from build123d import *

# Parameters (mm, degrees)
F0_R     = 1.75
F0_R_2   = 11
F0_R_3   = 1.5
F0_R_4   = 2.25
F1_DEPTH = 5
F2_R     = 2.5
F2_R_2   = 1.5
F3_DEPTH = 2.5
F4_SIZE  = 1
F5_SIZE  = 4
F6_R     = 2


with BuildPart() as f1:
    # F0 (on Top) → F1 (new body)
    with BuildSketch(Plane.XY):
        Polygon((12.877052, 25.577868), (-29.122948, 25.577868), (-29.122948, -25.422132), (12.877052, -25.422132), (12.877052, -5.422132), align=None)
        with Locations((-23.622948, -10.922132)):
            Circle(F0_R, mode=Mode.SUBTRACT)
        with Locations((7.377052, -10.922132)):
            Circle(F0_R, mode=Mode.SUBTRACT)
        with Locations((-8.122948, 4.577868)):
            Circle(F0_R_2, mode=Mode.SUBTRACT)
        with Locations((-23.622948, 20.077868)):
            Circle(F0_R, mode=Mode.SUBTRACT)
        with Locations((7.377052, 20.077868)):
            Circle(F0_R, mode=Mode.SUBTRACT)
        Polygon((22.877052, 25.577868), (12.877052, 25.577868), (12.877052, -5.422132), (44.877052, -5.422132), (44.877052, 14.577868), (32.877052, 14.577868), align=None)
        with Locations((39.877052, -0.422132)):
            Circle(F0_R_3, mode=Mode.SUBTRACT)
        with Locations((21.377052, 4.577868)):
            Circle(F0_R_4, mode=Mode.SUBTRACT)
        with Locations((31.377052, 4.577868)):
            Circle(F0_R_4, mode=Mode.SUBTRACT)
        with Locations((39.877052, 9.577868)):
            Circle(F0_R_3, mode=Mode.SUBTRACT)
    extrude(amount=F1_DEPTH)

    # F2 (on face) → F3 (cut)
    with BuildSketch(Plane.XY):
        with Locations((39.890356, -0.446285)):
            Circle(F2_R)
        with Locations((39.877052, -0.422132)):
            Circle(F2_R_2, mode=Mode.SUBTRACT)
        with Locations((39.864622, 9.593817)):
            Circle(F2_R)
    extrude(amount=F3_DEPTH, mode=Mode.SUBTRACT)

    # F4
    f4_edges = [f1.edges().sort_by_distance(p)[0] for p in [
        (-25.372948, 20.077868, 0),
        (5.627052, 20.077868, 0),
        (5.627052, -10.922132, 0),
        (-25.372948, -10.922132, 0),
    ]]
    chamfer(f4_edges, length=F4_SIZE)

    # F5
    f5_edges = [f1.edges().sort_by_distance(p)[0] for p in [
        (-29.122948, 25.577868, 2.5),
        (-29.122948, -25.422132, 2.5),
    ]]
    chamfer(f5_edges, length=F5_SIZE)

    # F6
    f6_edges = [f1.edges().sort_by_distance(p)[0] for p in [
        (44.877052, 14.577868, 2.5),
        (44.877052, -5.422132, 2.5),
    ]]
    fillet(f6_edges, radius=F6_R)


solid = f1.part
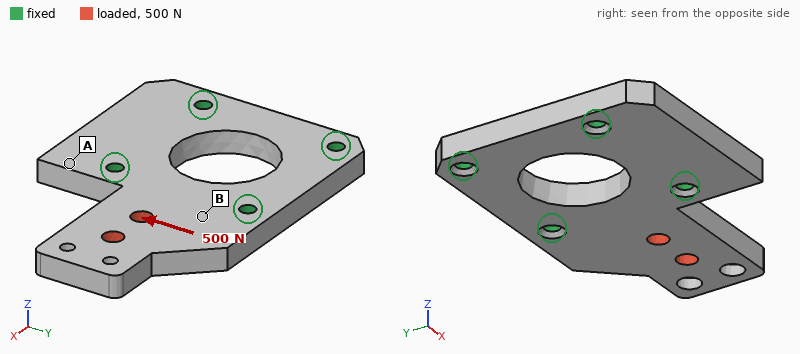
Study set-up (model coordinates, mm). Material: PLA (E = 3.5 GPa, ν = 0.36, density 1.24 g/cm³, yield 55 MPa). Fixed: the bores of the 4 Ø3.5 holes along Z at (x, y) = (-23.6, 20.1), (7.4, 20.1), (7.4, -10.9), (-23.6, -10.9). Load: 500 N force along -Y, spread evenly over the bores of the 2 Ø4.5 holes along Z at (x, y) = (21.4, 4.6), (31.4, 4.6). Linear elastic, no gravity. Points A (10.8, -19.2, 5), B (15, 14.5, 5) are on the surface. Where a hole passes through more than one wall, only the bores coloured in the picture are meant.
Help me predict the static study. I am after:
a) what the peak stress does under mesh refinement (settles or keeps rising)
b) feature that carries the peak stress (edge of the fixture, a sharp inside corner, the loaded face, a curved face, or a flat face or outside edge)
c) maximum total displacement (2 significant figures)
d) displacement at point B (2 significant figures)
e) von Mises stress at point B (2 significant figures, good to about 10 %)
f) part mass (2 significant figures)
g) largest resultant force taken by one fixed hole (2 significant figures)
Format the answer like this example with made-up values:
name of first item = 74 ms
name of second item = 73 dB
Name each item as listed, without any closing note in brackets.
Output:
what the peak stress does under mesh refinement = keeps rising
feature that carries the peak stress = edge of the fixture
maximum total displacement = 0.17 mm
displacement at point B = 0.032 mm
von Mises stress at point B = 6.6 MPa
part mass = 15 g
largest resultant force taken by one fixed hole = 390 N
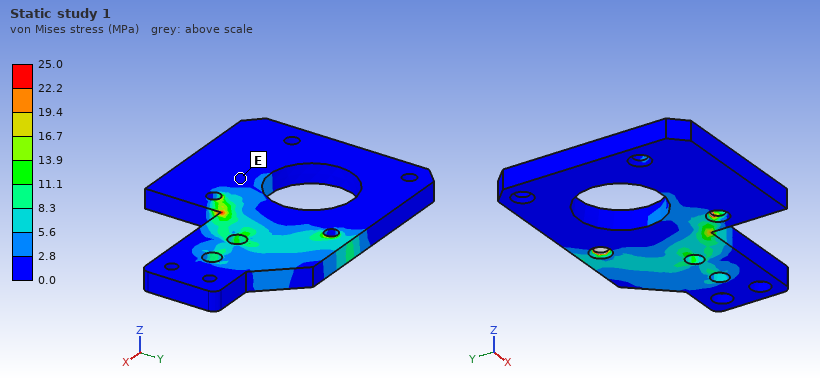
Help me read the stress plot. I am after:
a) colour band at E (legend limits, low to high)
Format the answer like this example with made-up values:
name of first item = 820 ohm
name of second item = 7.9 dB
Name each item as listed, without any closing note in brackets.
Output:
colour band at E = 0.0 to 2.8 MPa
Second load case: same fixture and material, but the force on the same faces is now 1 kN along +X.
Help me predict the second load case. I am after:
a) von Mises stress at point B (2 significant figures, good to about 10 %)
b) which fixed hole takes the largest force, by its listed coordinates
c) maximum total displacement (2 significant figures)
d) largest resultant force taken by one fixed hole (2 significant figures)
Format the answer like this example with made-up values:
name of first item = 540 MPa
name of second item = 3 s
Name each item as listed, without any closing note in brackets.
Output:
von Mises stress at point B = 7.4 MPa
which fixed hole takes the largest force, by its listed coordinates = (7.4, -10.9)
maximum total displacement = 0.17 mm
largest resultant force taken by one fixed hole = 520 N
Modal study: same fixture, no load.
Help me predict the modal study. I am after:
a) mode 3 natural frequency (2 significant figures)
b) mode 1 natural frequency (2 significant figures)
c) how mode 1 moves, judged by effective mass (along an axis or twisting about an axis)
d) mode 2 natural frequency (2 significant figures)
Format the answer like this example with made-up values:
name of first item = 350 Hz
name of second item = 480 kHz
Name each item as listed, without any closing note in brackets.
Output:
mode 3 natural frequency = 4200 Hz
mode 1 natural frequency = 1000 Hz
how mode 1 moves, judged by effective mass = along Z
mode 2 natural frequency = 3600 Hz
